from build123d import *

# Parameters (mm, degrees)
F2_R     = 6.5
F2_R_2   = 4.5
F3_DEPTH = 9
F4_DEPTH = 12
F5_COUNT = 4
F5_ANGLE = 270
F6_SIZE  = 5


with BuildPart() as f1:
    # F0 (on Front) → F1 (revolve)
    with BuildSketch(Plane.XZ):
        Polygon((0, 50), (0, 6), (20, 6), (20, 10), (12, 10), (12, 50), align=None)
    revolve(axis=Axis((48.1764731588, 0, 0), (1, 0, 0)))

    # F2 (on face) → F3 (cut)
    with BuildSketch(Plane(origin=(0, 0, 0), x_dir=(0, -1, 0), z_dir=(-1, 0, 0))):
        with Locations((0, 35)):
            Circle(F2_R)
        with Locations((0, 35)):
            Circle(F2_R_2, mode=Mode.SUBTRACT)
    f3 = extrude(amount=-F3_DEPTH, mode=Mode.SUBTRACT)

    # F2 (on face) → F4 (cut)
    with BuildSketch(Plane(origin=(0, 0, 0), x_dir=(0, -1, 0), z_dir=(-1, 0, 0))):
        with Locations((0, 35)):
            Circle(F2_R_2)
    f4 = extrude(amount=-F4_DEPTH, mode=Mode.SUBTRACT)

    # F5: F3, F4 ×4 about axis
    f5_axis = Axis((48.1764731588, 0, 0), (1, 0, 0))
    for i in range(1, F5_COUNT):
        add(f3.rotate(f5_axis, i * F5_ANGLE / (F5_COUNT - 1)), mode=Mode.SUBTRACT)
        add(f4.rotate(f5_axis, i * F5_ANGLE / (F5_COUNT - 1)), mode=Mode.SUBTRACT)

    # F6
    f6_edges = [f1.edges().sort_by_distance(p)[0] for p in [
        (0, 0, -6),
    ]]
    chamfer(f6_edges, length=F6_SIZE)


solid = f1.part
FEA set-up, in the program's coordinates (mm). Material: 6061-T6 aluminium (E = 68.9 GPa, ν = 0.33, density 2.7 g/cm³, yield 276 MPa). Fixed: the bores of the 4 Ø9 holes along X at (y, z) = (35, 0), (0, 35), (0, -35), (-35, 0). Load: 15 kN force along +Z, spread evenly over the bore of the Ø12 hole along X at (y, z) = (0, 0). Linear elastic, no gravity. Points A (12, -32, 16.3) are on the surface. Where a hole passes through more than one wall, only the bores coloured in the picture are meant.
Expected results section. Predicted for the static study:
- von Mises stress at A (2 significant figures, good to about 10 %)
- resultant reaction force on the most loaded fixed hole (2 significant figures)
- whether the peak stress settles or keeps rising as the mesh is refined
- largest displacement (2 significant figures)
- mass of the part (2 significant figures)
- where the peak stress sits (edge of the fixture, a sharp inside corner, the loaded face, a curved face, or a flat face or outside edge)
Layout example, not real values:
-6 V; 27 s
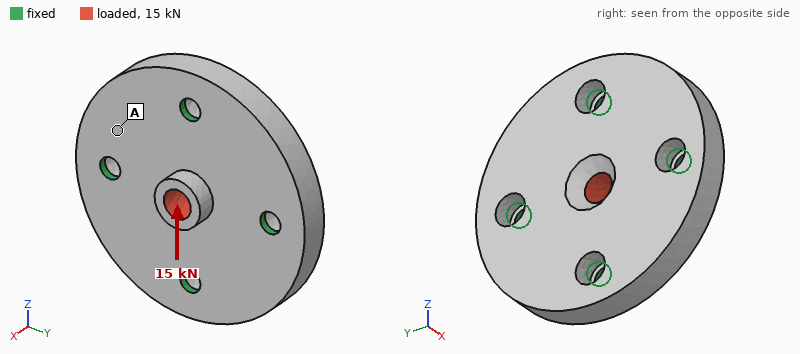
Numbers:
9.8 MPa; 4.0 kN; keeps rising; 44 µm; 240 g; edge of the fixture
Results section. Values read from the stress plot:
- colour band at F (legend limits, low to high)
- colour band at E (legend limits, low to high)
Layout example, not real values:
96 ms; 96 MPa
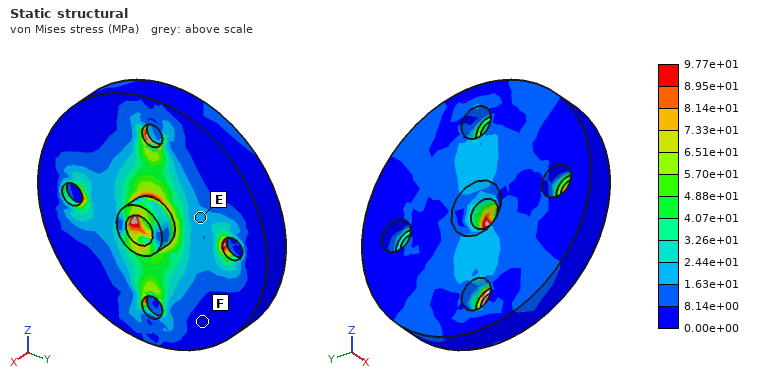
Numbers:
0.00e+00 to 8.14e+00 MPa; 1.63e+01 to 2.44e+01 MPa
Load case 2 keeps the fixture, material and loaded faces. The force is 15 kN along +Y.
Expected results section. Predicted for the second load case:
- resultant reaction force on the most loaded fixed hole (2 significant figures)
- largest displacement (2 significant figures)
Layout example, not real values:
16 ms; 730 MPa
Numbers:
4.0 kN; 43 µm
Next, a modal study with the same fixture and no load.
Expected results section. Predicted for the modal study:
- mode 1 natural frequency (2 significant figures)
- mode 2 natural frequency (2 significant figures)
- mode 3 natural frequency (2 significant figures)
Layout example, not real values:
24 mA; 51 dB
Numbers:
8300 Hz; 9300 Hz; 9300 Hz
